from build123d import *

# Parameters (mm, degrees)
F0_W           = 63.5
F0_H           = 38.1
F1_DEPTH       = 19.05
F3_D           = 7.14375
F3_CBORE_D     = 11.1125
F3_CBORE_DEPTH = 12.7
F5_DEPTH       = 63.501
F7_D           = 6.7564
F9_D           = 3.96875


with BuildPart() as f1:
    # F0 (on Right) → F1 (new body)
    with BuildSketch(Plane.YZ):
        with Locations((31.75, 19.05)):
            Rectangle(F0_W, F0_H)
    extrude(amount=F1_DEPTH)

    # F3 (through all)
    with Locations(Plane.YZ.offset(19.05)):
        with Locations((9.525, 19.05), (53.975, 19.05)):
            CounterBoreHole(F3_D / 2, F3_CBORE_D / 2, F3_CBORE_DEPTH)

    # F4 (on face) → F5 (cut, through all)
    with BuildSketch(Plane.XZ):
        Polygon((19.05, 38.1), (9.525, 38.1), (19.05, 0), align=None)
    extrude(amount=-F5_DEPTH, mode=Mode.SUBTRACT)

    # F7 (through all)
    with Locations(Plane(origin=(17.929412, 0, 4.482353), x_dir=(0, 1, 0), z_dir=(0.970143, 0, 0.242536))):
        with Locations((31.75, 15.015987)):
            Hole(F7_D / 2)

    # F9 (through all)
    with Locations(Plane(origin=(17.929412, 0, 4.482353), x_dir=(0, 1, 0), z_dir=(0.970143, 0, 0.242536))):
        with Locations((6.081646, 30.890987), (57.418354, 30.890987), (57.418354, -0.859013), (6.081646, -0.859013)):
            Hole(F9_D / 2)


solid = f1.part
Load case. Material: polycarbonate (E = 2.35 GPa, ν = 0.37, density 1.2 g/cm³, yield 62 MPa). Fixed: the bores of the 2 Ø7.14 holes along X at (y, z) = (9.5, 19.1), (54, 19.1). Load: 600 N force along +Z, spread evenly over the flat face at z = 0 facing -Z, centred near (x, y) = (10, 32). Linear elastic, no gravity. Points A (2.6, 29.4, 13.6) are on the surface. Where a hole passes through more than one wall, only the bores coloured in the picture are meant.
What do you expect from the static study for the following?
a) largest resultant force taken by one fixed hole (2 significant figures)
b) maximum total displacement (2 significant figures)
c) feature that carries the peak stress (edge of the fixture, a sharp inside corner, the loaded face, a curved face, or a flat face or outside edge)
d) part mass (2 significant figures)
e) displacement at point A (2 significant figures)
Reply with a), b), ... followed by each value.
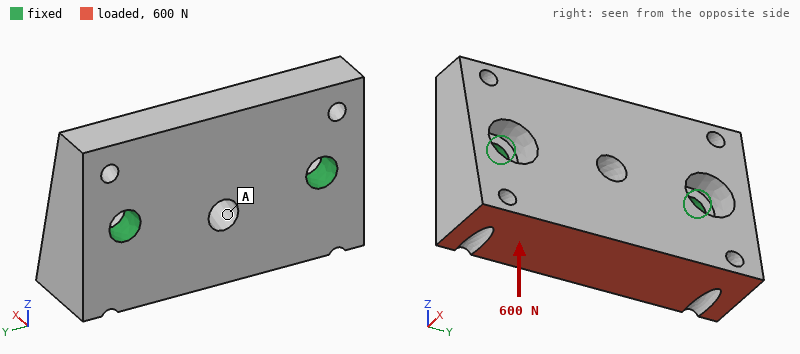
a) 300 N
b) 0.10 mm
c) the loaded face
d) 38 g
e) 0.022 mm
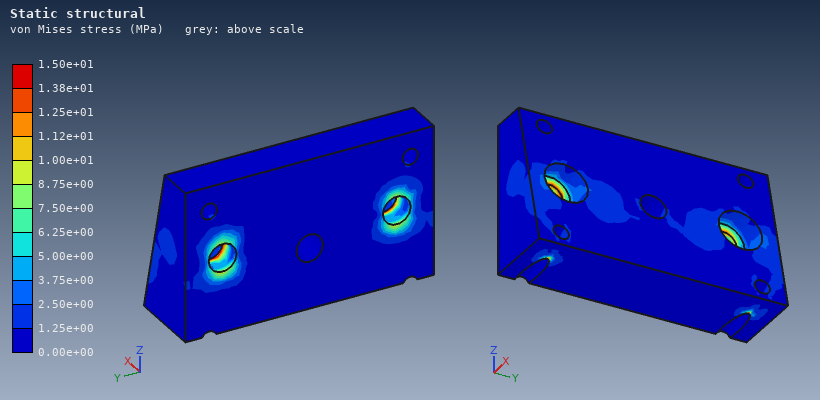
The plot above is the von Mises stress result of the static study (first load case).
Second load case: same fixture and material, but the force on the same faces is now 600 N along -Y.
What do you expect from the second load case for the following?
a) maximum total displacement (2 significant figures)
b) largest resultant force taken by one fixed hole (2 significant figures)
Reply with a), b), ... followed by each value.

a) 48 µm
b) 390 N
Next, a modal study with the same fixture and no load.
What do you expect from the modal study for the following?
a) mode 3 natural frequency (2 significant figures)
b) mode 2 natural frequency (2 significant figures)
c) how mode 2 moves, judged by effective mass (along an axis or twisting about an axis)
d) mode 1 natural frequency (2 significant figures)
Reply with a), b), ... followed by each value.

a) 4600 Hz
b) 4200 Hz
c) along X
d) 2300 Hz
